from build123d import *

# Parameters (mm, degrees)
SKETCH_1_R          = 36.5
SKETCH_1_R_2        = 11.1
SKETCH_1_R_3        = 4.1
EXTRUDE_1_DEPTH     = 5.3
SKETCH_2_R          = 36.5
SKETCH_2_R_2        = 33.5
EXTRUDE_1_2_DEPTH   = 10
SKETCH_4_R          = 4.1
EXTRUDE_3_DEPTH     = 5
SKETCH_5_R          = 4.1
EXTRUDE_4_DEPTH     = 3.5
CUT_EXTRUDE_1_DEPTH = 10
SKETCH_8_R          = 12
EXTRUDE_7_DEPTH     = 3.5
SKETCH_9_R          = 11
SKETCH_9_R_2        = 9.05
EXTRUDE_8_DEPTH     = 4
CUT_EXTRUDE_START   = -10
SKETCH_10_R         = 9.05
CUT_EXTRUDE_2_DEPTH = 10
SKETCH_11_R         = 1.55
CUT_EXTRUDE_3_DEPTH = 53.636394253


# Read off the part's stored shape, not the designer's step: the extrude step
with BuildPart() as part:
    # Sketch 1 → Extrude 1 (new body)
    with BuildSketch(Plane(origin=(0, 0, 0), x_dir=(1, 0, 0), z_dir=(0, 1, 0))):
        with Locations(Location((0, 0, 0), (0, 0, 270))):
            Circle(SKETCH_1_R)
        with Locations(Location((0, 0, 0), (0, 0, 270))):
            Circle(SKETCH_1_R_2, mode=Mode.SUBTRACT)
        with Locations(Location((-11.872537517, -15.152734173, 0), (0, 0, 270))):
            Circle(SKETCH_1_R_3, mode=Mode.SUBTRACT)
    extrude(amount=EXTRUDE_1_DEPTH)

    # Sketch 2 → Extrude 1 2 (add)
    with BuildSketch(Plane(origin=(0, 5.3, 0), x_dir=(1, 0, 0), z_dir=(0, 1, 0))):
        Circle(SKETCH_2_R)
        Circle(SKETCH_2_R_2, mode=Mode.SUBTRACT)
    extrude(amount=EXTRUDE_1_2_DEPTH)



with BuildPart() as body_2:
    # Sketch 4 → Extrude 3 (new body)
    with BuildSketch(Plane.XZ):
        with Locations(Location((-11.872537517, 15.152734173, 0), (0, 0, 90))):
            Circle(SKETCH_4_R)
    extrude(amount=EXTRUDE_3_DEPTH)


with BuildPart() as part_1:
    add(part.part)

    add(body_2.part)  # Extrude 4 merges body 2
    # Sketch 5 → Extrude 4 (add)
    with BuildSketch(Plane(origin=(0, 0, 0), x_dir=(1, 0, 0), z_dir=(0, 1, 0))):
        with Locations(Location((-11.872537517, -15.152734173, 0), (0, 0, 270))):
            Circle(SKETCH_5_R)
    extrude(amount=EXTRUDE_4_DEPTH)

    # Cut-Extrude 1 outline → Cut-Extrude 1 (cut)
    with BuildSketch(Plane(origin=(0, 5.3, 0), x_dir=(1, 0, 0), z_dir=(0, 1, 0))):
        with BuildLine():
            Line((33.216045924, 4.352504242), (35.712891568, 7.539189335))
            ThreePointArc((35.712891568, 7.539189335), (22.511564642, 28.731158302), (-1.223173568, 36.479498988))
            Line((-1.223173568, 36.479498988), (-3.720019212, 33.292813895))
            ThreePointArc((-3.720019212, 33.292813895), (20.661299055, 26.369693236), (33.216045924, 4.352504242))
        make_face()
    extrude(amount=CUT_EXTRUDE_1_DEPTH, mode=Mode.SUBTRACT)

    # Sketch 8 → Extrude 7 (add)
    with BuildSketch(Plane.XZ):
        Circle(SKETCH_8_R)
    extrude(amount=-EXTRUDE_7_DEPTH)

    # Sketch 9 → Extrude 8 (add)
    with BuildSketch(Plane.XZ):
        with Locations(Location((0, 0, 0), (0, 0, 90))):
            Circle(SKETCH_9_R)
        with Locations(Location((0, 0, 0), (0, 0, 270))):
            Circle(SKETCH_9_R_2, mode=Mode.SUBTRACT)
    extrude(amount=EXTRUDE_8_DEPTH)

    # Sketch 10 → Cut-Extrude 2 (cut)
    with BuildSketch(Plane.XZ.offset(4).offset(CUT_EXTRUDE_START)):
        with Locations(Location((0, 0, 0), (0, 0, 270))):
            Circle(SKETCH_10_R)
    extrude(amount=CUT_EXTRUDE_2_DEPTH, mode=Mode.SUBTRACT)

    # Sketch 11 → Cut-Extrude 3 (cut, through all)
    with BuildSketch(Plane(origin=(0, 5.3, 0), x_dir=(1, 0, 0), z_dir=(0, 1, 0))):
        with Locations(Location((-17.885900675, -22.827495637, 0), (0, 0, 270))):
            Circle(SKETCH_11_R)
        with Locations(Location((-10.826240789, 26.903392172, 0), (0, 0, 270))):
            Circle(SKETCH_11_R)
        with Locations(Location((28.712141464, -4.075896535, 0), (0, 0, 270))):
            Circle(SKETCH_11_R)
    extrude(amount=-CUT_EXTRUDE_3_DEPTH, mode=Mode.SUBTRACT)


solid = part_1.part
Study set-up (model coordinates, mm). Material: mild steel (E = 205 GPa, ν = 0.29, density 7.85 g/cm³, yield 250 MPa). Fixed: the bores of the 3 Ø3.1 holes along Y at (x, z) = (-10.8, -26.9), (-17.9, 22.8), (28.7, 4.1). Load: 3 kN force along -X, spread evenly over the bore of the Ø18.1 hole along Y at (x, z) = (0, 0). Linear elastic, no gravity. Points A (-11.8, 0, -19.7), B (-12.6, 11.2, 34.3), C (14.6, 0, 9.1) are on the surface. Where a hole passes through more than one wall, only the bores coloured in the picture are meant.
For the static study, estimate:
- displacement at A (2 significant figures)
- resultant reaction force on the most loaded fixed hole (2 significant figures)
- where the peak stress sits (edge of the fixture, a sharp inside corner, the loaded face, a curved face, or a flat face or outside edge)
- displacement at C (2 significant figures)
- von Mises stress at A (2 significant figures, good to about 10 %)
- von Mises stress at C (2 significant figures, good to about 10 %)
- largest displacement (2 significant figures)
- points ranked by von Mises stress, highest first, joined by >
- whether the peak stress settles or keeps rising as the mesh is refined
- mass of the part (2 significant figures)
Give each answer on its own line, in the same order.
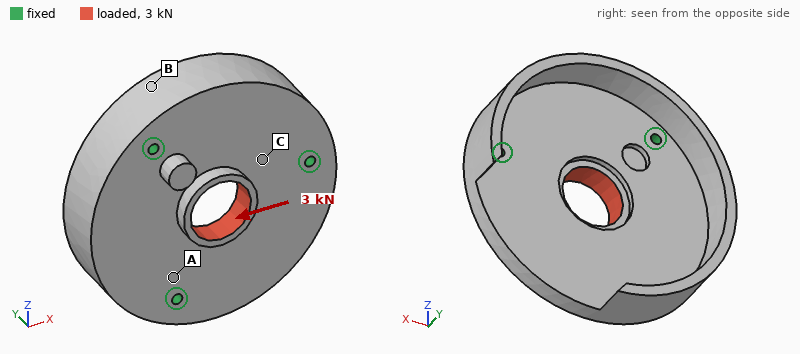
0.95 µm
1.0 kN
edge of the fixture
1.2 µm
7.6 MPa
15 MPa
4.7 µm
C > A > B
keeps rising
210 g
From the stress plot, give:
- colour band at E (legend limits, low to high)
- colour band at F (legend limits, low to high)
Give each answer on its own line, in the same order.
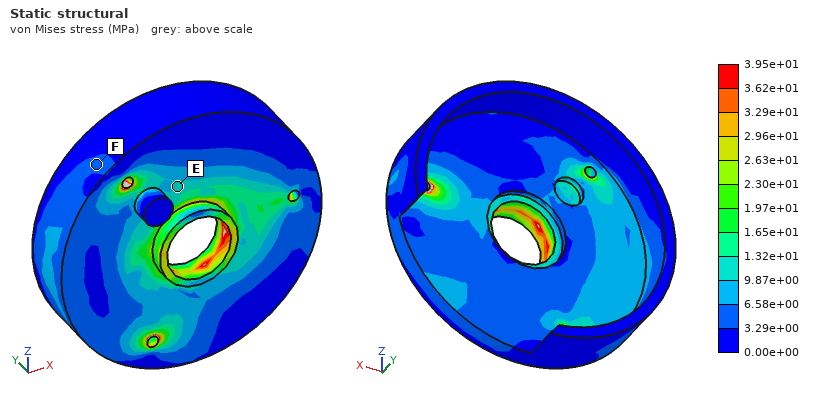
9.87e+00 to 1.32e+01 MPa
3.29e+00 to 6.58e+00 MPa
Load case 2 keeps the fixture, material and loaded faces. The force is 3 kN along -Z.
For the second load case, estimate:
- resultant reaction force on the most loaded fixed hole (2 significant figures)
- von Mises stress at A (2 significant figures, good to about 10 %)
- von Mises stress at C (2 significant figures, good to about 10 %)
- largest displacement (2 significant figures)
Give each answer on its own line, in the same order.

1.0 kN
15 MPa
9.1 MPa
4.6 µm
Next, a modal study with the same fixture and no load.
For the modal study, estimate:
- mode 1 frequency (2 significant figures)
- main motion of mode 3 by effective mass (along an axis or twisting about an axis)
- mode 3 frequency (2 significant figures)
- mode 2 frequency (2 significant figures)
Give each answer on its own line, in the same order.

5600 Hz
along Y
8300 Hz
6300 Hz
